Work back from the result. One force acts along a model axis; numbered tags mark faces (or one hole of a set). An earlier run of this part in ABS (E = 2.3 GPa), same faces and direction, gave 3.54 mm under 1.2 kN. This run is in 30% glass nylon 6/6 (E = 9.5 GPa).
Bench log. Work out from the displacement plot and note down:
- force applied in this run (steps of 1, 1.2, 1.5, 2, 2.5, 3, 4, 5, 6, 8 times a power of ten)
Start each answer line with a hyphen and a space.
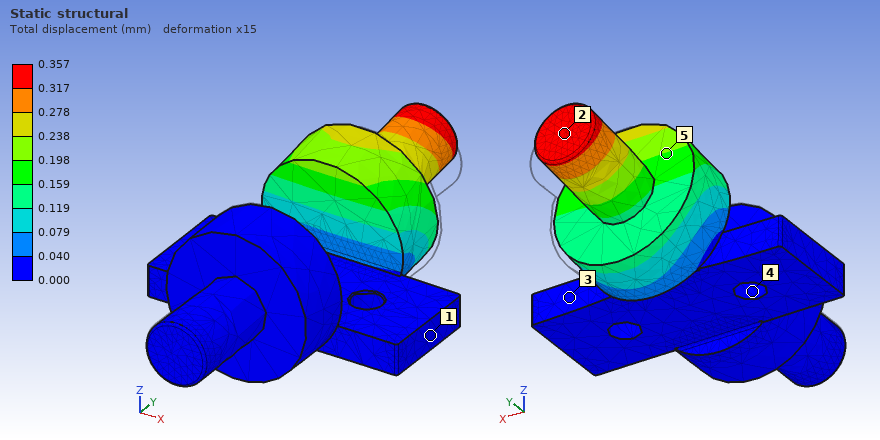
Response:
- 500 N
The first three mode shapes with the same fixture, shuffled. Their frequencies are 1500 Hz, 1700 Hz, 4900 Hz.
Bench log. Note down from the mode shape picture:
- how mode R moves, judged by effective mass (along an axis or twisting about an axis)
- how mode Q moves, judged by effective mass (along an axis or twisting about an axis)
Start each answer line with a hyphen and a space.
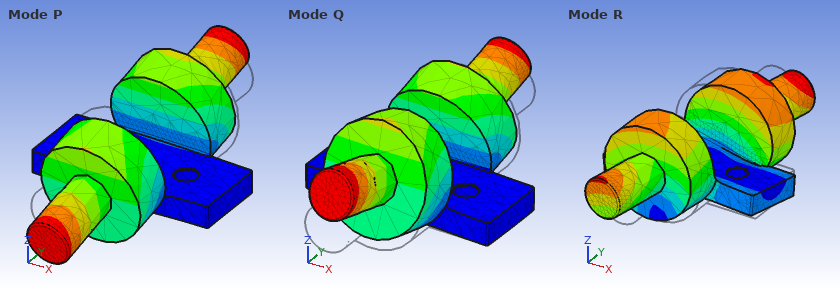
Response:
- twisting about Z
- along Z
